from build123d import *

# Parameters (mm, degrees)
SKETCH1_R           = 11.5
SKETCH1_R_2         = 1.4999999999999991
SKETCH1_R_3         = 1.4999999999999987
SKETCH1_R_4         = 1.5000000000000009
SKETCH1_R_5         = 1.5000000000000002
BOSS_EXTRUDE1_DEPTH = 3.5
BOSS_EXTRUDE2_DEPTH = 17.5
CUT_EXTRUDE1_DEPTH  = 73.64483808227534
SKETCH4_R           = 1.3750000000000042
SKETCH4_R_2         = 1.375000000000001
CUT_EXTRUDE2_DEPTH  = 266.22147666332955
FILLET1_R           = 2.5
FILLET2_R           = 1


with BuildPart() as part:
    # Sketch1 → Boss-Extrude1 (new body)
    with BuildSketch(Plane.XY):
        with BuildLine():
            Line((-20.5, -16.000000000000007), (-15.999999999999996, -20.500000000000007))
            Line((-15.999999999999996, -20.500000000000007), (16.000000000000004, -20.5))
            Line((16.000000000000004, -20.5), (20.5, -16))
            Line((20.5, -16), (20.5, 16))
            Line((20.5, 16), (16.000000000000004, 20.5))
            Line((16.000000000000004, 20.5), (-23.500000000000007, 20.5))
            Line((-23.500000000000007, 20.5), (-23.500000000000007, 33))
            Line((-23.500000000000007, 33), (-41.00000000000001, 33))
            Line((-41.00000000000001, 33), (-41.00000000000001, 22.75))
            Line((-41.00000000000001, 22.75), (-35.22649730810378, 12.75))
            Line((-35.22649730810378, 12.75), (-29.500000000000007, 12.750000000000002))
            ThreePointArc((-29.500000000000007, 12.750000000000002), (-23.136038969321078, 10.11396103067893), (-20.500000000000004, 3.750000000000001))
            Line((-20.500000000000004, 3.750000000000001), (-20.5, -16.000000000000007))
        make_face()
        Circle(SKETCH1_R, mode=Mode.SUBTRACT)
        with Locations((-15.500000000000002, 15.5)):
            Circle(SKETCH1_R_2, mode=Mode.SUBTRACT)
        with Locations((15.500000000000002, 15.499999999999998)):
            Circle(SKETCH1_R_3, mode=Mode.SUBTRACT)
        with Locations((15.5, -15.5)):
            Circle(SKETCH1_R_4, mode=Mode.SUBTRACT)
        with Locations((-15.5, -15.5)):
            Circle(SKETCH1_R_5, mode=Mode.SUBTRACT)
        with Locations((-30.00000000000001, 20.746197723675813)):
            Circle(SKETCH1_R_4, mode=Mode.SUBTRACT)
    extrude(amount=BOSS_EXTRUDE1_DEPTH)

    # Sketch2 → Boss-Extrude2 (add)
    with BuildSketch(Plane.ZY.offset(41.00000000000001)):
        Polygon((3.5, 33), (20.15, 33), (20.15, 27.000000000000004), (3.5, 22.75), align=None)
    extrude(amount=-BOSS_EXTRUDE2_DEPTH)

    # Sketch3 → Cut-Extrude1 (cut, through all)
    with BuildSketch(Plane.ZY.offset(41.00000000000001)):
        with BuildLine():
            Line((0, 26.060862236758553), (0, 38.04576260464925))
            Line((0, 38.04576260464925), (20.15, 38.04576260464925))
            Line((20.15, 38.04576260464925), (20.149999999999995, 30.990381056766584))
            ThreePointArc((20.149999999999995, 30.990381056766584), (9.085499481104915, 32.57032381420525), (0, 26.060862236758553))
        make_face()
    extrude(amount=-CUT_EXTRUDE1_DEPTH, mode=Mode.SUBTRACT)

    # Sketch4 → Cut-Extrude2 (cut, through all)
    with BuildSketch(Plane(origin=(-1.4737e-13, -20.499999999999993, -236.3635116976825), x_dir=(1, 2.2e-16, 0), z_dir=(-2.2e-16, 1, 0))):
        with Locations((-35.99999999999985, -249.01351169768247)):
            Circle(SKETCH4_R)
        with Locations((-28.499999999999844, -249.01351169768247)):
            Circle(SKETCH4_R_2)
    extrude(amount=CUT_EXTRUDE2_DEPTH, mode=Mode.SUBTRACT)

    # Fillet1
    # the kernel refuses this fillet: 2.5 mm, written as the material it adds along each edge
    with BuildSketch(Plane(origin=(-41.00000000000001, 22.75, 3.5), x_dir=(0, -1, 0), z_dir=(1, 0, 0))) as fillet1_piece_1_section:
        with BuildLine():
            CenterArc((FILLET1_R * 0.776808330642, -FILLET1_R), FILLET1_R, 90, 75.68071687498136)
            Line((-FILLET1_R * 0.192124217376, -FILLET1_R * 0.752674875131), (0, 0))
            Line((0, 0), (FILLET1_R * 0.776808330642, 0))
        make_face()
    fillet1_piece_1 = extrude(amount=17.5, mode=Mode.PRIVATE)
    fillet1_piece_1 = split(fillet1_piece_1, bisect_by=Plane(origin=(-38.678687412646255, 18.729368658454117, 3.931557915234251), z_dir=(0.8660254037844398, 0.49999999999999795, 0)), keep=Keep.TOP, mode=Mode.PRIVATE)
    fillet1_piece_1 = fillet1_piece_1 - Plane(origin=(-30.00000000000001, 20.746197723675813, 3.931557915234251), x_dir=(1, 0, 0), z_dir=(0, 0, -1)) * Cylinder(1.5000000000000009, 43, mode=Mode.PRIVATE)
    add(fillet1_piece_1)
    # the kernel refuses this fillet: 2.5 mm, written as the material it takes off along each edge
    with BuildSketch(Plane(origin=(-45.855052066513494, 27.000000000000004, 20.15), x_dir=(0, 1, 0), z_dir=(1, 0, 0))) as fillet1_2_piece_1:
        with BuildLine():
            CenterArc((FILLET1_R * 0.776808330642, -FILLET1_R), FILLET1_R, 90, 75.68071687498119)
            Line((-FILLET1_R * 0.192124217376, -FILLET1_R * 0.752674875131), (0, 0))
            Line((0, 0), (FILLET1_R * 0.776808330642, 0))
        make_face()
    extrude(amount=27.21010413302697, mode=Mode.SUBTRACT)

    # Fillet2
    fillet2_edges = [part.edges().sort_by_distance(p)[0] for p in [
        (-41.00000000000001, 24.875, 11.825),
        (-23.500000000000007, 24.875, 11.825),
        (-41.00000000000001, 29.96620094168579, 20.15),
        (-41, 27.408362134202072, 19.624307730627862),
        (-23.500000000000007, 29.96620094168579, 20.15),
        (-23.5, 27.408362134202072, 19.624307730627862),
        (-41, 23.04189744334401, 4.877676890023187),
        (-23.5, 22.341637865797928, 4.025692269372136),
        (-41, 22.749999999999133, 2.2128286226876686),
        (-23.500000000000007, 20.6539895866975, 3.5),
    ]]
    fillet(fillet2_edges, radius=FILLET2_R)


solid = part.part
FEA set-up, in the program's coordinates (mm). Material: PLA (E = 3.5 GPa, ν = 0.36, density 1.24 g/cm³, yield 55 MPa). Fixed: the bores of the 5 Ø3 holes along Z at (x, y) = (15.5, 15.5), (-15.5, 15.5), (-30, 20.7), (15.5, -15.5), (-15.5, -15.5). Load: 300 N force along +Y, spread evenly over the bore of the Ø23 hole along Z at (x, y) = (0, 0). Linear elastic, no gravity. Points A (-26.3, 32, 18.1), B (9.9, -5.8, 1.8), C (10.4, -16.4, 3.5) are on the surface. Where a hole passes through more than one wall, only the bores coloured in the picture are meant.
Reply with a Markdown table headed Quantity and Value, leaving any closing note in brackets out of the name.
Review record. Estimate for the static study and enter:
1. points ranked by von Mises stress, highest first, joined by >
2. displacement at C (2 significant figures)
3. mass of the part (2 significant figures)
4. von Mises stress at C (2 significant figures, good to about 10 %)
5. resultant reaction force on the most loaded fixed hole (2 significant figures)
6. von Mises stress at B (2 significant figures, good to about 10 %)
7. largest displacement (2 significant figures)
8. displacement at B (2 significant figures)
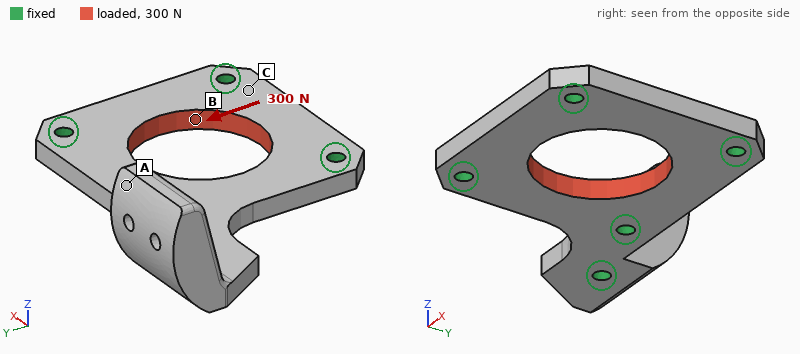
| Quantity | Value |
|---|---|
| points ranked by von Mises stress, highest first, joined by > | B > C > A |
| displacement at C | 6.8 µm |
| mass of the part | 8.9 g |
| von Mises stress at C | 1.6 MPa |
| resultant reaction force on the most loaded fixed hole | 77 N |
| von Mises stress at B | 3.1 MPa |
| largest displacement | 18 µm |
| displacement at B | 8.7 µm |
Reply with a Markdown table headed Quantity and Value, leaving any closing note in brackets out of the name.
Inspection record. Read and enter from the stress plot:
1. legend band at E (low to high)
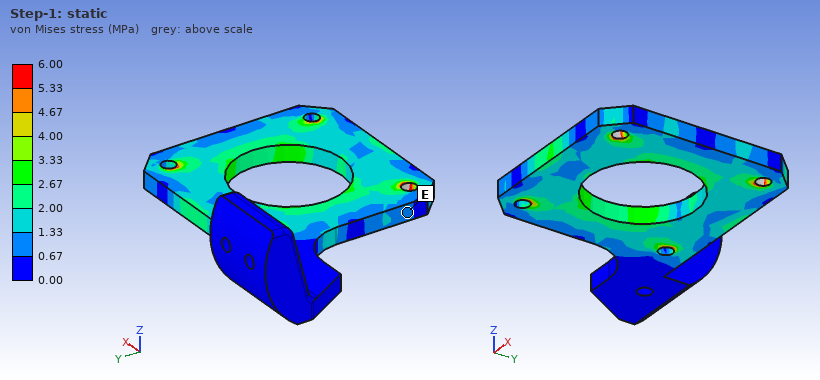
| Quantity | Value |
|---|---|
| legend band at E | 0.67 to 1.33 MPa |
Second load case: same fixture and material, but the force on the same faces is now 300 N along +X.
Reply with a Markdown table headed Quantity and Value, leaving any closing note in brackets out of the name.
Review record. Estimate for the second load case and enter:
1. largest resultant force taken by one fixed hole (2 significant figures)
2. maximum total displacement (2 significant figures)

| Quantity | Value |
|---|---|
| largest resultant force taken by one fixed hole | 76 N |
| maximum total displacement | 19 µm |
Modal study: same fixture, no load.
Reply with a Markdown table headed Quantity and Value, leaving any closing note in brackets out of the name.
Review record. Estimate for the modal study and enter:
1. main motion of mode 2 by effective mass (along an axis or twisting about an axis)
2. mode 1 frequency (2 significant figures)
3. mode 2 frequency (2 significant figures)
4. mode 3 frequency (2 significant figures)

| Quantity | Value |
|---|---|
| main motion of mode 2 by effective mass | along X |
| mode 1 frequency | 2000 Hz |
| mode 2 frequency | 2500 Hz |
| mode 3 frequency | 5500 Hz |
